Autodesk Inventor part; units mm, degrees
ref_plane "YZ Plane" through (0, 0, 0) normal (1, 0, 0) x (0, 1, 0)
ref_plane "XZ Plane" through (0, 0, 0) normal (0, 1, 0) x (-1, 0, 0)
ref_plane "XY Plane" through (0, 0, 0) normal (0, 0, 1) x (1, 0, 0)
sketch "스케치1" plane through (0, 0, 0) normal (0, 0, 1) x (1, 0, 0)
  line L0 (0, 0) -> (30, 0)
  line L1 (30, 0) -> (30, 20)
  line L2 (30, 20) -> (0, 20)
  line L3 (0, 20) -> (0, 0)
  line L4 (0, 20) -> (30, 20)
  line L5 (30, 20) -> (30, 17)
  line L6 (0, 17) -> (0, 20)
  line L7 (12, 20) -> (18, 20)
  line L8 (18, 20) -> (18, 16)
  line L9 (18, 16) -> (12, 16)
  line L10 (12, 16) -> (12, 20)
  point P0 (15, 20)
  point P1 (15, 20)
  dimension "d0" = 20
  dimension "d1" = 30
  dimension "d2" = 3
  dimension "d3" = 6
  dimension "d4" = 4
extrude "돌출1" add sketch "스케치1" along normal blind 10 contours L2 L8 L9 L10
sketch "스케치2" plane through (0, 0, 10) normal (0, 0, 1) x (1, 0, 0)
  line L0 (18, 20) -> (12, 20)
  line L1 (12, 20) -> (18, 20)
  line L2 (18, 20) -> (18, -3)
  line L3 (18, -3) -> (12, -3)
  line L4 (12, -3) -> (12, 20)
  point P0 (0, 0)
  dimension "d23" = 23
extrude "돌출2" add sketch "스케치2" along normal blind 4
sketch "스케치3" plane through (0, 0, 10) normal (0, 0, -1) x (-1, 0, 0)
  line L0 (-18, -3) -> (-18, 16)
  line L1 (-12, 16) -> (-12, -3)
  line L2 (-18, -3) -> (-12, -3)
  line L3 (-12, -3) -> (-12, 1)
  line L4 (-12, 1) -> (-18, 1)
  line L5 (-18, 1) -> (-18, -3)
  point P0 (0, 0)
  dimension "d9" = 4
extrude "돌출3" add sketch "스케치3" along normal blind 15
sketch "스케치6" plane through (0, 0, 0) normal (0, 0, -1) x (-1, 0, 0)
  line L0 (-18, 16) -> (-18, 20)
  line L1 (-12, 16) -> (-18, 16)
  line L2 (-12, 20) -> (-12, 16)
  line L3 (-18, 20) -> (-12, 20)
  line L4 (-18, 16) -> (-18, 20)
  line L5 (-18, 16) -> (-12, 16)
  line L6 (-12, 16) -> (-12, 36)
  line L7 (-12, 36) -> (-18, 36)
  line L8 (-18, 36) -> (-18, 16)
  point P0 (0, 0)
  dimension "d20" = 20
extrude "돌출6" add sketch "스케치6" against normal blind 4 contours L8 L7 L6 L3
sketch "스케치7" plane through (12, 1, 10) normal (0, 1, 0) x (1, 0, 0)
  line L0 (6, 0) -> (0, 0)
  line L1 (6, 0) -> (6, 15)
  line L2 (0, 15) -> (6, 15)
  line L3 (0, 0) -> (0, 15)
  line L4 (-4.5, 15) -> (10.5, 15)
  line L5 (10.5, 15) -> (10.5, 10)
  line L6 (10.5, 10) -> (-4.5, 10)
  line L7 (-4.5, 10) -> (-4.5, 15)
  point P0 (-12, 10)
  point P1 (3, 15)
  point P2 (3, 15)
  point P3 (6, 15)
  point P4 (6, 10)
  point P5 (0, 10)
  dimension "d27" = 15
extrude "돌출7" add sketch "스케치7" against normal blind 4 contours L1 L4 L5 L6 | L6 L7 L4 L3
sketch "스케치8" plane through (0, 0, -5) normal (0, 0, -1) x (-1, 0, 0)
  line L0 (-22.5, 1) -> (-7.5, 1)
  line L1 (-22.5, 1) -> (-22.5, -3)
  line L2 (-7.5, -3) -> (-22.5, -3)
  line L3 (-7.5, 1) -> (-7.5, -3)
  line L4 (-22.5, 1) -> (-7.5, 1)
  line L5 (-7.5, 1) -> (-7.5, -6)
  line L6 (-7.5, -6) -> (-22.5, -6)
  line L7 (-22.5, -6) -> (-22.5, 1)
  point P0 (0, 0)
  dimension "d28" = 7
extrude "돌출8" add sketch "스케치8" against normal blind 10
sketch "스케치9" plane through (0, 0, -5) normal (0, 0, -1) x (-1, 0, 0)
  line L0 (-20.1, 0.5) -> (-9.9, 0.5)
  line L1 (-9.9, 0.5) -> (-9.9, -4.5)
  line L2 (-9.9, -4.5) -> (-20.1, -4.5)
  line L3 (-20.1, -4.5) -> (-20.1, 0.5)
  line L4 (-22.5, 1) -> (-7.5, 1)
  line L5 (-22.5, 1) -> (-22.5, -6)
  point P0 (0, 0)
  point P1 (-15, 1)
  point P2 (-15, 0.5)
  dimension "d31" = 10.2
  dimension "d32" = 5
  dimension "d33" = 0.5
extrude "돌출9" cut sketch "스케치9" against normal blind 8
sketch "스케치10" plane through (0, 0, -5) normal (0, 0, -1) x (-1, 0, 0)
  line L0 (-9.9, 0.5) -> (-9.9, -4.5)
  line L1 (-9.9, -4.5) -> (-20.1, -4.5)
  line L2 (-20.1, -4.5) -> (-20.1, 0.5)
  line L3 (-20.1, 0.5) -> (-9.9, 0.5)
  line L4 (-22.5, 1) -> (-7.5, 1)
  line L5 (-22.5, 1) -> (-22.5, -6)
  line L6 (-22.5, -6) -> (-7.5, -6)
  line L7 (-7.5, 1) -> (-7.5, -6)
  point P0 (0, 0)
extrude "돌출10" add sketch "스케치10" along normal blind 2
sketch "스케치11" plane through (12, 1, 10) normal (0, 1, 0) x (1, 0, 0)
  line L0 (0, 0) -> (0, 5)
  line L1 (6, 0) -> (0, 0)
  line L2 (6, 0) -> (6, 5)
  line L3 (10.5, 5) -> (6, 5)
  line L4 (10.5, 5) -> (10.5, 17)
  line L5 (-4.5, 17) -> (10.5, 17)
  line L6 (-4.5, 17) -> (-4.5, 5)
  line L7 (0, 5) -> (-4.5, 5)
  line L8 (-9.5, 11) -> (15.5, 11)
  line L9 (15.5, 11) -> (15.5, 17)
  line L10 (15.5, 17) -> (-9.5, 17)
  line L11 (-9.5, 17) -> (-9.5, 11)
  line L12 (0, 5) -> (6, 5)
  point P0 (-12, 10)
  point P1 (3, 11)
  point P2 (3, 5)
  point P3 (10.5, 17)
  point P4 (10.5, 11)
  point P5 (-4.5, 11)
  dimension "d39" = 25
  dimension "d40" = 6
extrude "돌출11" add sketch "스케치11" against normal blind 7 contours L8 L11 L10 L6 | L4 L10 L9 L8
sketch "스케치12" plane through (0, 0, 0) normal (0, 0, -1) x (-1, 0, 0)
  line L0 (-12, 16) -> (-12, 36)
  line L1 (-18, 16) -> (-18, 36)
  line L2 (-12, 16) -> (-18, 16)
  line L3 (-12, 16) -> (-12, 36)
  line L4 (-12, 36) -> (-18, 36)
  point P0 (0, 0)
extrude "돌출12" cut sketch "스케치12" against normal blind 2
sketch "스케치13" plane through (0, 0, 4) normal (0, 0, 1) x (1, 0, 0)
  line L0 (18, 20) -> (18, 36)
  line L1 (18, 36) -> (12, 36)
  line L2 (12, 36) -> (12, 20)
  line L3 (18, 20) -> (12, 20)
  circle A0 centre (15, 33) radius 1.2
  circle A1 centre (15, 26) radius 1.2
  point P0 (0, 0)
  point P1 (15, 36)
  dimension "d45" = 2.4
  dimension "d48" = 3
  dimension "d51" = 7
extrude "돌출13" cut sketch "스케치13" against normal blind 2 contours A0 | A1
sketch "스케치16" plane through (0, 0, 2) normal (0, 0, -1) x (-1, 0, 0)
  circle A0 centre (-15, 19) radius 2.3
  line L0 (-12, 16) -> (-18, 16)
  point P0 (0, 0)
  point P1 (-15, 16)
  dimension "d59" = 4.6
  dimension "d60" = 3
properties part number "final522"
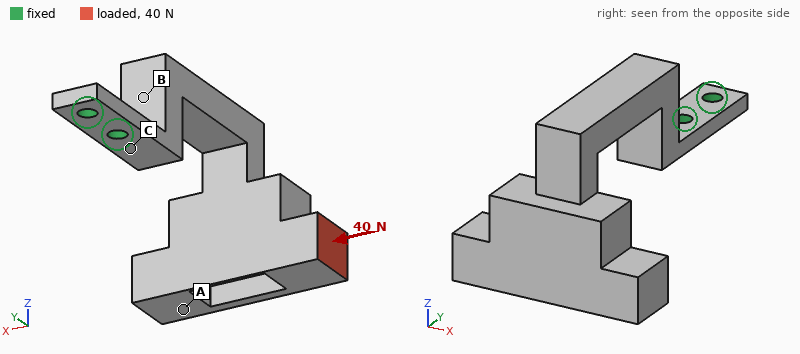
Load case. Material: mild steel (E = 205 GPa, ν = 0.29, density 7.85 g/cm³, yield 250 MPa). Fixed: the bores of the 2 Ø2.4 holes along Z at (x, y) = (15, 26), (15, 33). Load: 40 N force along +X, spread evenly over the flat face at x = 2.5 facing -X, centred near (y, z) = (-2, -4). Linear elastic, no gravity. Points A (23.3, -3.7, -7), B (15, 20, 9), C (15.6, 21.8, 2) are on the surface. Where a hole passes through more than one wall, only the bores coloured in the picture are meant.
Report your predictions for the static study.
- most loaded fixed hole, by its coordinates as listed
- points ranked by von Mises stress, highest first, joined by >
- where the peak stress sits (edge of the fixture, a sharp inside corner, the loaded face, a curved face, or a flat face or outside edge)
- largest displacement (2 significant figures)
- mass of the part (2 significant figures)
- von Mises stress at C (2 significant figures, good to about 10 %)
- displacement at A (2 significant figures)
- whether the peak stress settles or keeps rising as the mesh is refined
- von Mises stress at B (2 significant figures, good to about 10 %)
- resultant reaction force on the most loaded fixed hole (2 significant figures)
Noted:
(15, 26)
C > B > A
edge of the fixture
0.14 mm
17 g
75 MPa
0.13 mm
keeps rising
55 MPa
94 N
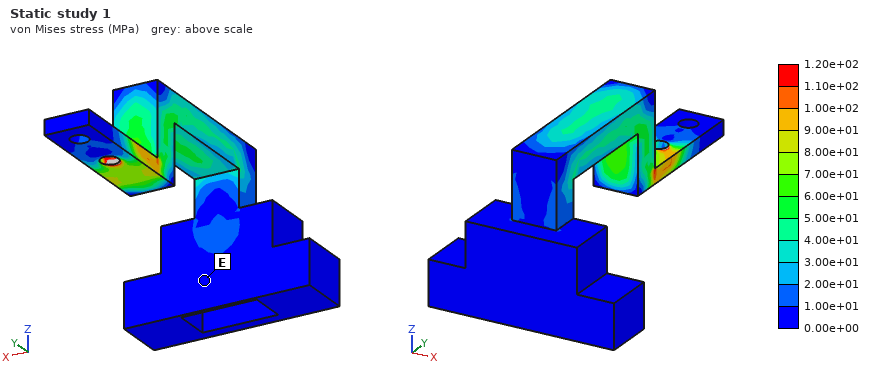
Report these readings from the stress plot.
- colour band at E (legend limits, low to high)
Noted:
0.00e+00 to 1.00e+01 MPa
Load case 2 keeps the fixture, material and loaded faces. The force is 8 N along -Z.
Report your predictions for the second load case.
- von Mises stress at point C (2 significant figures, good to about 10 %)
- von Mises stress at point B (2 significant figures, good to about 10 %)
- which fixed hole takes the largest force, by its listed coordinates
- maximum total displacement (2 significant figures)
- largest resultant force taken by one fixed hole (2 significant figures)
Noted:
50 MPa
9.3 MPa
(15, 26)
67 µm
10 N
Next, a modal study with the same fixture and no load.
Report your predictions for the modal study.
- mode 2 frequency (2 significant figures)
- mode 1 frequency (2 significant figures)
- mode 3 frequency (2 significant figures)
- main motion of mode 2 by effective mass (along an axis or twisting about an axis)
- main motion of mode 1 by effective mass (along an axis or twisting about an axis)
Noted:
1000 Hz
590 Hz
1900 Hz
along X
along Z
